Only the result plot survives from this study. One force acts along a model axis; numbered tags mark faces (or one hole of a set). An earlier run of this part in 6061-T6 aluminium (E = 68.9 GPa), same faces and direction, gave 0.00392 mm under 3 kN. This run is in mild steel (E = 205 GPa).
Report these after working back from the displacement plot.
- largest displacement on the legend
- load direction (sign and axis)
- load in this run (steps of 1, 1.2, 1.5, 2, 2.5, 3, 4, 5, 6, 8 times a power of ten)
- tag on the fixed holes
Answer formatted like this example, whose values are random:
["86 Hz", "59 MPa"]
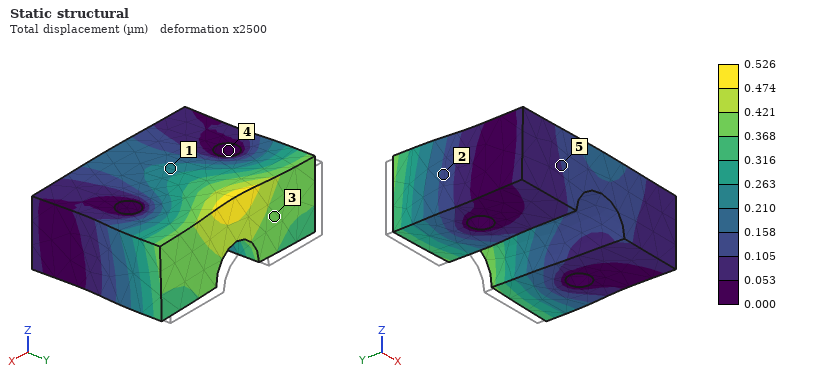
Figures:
["0.526 µm", "-Y", "1.2 kN", "4"]
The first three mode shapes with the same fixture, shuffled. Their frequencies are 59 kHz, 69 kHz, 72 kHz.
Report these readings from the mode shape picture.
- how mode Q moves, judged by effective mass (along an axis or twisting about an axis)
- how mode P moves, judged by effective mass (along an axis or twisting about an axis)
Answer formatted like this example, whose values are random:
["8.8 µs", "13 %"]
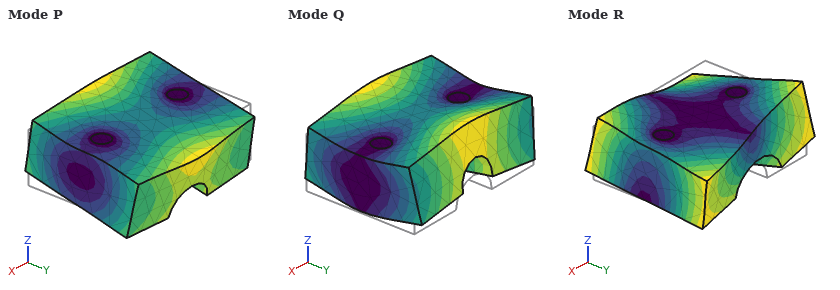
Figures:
["along Z", "twisting about X"]
